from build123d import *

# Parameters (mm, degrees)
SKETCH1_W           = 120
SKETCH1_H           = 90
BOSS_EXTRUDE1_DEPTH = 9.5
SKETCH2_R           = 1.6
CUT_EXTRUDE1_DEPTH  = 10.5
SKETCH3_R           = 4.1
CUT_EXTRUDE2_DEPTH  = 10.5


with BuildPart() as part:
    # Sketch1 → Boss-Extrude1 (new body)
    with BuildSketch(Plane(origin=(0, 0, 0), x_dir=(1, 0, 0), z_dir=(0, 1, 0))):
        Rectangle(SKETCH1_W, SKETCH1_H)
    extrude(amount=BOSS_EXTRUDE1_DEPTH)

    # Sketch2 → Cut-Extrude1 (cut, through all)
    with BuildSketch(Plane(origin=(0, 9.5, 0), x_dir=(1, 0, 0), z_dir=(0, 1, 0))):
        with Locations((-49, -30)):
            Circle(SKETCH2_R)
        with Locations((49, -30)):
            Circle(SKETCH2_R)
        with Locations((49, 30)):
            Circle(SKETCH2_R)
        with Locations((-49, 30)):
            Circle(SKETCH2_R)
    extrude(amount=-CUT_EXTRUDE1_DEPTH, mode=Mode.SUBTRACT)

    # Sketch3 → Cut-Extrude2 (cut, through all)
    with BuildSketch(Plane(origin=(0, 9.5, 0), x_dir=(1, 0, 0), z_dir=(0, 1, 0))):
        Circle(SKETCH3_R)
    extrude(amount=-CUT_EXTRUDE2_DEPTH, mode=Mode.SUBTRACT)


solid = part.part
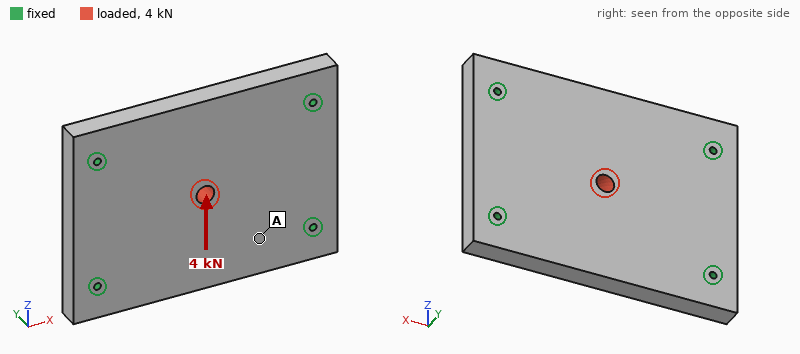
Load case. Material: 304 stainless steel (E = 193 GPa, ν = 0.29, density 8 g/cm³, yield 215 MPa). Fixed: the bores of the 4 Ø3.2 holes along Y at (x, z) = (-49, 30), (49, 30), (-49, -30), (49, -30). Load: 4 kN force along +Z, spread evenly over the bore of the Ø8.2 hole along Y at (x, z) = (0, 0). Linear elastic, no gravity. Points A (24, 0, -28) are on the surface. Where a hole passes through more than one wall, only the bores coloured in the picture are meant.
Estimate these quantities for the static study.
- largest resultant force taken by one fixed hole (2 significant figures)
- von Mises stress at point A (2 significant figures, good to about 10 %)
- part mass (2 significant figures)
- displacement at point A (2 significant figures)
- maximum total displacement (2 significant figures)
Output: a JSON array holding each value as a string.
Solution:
["1.2 kN", "4.1 MPa", "810 g", "1.4 µm", "2.9 µm"]
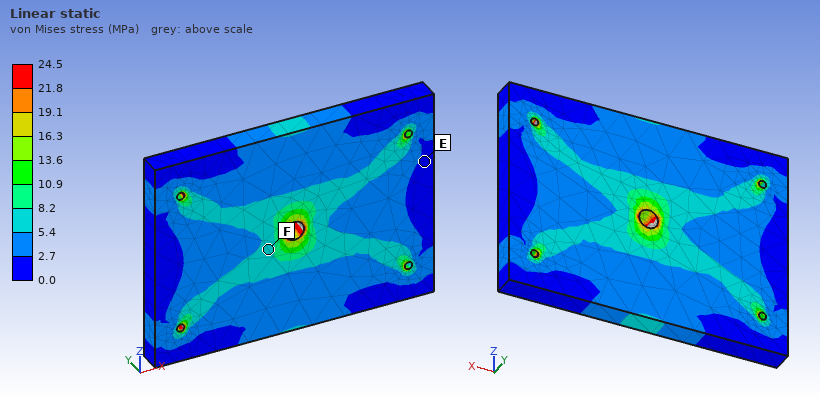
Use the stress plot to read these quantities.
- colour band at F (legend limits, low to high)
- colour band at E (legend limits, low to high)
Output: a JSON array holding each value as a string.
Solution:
["5.4 to 8.2 MPa", "0.0 to 2.7 MPa"]
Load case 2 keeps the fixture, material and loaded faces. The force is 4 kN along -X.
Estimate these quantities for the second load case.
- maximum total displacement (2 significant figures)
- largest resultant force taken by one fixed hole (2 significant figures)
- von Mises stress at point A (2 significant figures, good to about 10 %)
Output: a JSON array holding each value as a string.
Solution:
["2.0 µm", "1.0 kN", "3.0 MPa"]
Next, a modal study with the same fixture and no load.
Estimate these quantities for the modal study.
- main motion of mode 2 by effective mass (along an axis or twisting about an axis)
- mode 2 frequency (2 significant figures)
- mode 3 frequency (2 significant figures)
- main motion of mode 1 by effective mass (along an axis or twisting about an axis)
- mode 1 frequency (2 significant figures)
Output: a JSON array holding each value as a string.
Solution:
["twisting about X", "5000 Hz", "7800 Hz", "along Y", "3600 Hz"]
